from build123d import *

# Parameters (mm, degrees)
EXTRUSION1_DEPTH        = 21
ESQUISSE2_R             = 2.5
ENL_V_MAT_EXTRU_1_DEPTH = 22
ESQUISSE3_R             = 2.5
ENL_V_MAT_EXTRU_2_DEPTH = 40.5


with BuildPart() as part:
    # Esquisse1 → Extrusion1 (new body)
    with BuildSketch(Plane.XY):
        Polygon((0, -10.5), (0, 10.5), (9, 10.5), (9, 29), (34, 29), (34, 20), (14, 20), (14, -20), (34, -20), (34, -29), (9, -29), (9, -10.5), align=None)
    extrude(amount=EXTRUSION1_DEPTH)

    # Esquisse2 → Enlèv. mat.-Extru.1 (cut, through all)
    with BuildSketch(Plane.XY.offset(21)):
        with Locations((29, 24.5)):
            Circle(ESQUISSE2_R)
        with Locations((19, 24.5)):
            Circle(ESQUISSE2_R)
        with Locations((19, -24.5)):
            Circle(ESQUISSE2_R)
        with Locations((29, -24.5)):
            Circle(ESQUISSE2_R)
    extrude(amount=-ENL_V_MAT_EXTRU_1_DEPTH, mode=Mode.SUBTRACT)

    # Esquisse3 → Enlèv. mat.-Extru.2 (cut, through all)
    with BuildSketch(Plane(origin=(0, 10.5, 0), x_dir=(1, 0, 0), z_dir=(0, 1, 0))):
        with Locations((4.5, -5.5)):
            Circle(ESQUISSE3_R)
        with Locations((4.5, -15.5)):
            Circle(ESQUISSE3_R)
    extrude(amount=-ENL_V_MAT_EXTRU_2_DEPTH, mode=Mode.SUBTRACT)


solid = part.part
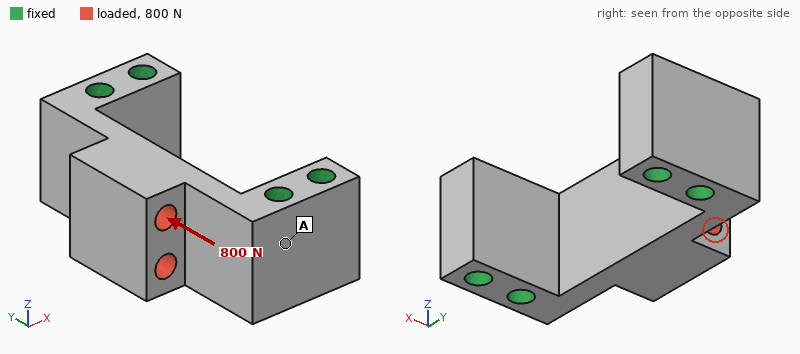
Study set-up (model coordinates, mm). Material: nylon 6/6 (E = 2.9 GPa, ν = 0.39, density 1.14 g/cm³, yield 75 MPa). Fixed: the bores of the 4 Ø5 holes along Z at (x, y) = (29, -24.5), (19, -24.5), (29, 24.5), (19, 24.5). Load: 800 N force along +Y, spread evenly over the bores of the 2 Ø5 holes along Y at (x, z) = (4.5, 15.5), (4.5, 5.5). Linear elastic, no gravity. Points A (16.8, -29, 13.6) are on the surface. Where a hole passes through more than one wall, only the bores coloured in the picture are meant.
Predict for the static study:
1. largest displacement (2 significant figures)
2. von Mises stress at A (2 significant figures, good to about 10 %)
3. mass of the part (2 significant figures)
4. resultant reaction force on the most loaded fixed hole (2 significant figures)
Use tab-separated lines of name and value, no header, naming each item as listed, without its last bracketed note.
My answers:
largest displacement	92 µm
von Mises stress at A	2.3 MPa
mass of the part	17 g
resultant reaction force on the most loaded fixed hole	450 N
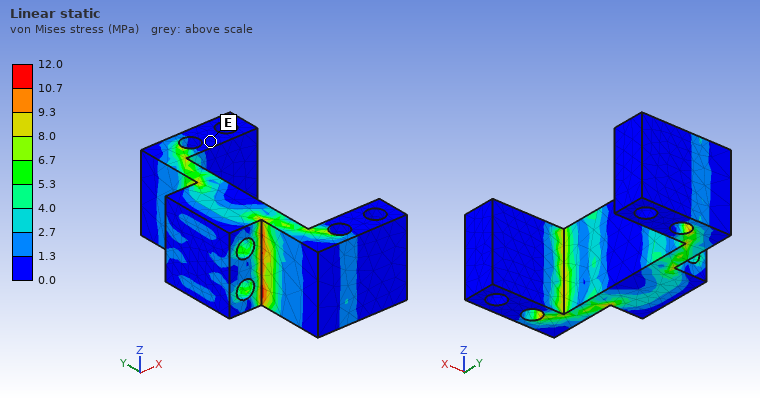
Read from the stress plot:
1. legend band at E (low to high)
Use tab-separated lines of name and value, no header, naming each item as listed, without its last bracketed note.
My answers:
legend band at E	0.0 to 1.3 MPa
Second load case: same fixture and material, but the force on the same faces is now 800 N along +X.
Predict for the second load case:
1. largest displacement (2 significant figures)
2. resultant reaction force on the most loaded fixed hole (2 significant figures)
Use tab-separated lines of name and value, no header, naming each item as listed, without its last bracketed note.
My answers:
largest displacement	0.23 mm
resultant reaction force on the most loaded fixed hole	540 N
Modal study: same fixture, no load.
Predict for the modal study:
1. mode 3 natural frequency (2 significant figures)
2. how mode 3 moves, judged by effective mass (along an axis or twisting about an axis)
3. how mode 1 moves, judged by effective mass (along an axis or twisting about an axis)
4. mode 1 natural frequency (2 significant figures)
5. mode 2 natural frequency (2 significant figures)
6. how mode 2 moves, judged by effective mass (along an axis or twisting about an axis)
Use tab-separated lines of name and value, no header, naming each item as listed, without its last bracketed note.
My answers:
mode 3 natural frequency	5900 Hz
how mode 3 moves, judged by effective mass	along Z
how mode 1 moves, judged by effective mass	along Z
mode 1 natural frequency	3300 Hz
mode 2 natural frequency	3700 Hz
how mode 2 moves, judged by effective mass	along X
